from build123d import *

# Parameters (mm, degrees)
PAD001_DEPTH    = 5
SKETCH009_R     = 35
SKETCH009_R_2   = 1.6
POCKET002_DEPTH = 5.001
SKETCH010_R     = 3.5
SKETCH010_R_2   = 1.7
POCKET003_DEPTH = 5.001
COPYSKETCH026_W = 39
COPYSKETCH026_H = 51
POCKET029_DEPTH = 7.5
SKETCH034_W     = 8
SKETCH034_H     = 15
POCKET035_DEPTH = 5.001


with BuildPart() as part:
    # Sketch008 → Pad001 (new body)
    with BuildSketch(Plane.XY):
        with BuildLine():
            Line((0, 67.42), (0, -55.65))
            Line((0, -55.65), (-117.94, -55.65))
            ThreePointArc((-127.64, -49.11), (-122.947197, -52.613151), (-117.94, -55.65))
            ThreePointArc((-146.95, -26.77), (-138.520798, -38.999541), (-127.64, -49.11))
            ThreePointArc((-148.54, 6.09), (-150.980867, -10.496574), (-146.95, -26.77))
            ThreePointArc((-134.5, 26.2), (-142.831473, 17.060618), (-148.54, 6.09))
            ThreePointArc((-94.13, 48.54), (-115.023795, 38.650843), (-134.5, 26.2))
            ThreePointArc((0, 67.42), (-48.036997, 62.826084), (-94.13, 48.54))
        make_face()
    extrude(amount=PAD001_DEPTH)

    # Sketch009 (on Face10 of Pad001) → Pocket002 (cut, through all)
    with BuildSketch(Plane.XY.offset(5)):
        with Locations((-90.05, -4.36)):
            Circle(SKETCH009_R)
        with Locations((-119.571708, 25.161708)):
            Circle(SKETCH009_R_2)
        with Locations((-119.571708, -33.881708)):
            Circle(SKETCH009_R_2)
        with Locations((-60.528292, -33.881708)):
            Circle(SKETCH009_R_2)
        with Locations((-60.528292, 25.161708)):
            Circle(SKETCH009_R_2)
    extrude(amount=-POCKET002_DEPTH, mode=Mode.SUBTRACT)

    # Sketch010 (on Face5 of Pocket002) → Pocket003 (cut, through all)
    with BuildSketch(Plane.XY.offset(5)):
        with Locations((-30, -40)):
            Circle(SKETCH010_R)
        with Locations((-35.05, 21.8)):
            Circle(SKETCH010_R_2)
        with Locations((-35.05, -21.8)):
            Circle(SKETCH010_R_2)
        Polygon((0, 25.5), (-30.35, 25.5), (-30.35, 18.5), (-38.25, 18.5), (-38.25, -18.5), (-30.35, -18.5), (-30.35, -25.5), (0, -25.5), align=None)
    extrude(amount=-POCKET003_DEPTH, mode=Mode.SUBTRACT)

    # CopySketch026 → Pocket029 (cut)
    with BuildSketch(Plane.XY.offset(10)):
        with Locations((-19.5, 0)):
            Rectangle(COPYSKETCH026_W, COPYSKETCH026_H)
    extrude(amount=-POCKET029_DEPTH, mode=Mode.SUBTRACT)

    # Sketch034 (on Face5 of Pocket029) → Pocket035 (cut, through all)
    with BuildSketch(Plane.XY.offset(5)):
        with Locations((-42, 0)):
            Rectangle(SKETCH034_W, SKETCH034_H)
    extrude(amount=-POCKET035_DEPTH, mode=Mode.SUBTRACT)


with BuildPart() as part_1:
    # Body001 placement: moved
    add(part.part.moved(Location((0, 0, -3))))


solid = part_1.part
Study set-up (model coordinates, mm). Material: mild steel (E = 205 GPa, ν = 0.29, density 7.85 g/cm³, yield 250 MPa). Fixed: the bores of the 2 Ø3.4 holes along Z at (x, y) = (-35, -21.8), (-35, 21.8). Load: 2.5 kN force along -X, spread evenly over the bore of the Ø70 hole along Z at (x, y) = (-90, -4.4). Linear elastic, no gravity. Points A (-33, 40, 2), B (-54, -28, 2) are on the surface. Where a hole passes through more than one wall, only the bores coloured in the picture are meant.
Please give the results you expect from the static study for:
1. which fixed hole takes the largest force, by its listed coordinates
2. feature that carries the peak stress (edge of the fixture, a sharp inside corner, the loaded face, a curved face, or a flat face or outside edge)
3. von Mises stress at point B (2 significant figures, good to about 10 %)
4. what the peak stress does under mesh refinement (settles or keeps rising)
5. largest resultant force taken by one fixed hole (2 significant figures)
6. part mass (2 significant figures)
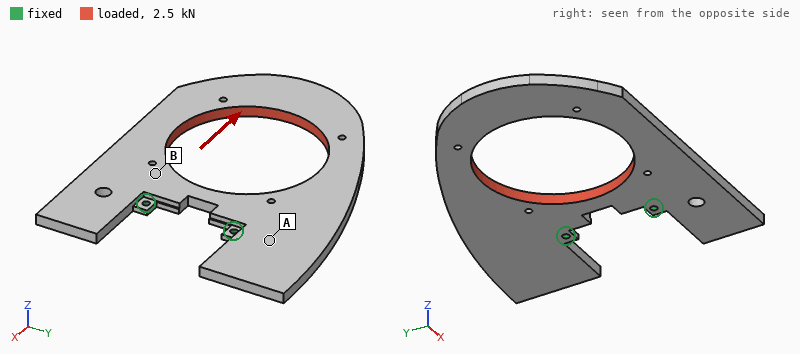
(-35, -21.8)
edge of the fixture
16 MPa
keeps rising
1.5 kN
380 g
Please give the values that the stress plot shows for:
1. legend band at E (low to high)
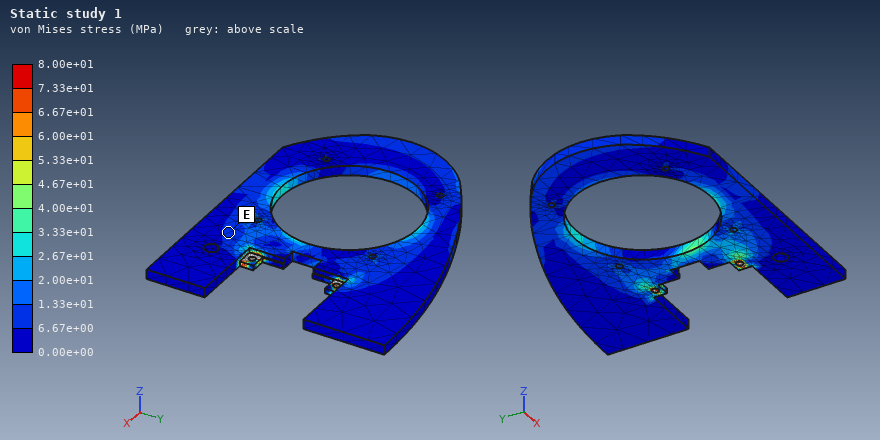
6.67e+00 to 1.33e+01 MPa
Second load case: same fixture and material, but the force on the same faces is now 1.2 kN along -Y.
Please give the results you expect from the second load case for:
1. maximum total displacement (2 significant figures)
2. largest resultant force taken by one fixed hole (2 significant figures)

79 µm
1.5 kN
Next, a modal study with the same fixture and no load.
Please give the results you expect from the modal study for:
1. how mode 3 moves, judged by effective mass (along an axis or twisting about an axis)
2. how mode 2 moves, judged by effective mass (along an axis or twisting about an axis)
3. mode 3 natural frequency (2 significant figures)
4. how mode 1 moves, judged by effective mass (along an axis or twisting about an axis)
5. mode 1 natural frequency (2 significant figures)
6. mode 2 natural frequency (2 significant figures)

along Z
twisting about X
980 Hz
along Z
210 Hz
600 Hz
